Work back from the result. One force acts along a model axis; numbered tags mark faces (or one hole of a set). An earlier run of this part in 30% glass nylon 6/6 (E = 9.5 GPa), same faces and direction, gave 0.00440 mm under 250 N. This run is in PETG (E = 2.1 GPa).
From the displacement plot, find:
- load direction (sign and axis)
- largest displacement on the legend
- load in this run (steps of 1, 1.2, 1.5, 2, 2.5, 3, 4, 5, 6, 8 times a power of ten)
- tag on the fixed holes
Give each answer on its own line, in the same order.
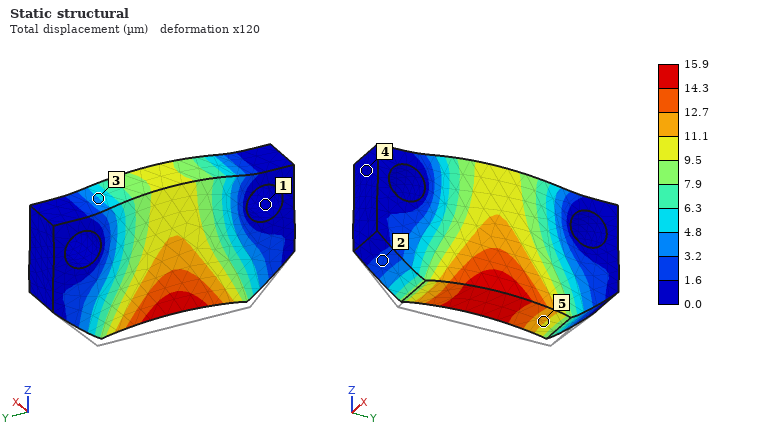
+Z
15.9 µm
200 N
1
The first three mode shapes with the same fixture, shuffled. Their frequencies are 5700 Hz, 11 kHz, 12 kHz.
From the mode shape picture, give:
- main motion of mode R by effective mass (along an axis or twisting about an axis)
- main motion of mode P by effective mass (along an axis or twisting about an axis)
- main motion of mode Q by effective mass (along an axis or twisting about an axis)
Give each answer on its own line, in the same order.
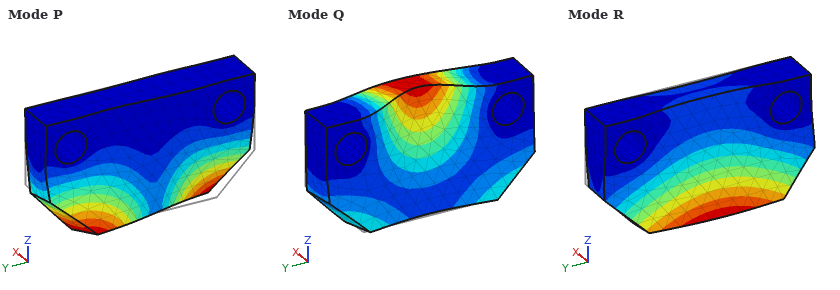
along X
twisting about Z
along X
